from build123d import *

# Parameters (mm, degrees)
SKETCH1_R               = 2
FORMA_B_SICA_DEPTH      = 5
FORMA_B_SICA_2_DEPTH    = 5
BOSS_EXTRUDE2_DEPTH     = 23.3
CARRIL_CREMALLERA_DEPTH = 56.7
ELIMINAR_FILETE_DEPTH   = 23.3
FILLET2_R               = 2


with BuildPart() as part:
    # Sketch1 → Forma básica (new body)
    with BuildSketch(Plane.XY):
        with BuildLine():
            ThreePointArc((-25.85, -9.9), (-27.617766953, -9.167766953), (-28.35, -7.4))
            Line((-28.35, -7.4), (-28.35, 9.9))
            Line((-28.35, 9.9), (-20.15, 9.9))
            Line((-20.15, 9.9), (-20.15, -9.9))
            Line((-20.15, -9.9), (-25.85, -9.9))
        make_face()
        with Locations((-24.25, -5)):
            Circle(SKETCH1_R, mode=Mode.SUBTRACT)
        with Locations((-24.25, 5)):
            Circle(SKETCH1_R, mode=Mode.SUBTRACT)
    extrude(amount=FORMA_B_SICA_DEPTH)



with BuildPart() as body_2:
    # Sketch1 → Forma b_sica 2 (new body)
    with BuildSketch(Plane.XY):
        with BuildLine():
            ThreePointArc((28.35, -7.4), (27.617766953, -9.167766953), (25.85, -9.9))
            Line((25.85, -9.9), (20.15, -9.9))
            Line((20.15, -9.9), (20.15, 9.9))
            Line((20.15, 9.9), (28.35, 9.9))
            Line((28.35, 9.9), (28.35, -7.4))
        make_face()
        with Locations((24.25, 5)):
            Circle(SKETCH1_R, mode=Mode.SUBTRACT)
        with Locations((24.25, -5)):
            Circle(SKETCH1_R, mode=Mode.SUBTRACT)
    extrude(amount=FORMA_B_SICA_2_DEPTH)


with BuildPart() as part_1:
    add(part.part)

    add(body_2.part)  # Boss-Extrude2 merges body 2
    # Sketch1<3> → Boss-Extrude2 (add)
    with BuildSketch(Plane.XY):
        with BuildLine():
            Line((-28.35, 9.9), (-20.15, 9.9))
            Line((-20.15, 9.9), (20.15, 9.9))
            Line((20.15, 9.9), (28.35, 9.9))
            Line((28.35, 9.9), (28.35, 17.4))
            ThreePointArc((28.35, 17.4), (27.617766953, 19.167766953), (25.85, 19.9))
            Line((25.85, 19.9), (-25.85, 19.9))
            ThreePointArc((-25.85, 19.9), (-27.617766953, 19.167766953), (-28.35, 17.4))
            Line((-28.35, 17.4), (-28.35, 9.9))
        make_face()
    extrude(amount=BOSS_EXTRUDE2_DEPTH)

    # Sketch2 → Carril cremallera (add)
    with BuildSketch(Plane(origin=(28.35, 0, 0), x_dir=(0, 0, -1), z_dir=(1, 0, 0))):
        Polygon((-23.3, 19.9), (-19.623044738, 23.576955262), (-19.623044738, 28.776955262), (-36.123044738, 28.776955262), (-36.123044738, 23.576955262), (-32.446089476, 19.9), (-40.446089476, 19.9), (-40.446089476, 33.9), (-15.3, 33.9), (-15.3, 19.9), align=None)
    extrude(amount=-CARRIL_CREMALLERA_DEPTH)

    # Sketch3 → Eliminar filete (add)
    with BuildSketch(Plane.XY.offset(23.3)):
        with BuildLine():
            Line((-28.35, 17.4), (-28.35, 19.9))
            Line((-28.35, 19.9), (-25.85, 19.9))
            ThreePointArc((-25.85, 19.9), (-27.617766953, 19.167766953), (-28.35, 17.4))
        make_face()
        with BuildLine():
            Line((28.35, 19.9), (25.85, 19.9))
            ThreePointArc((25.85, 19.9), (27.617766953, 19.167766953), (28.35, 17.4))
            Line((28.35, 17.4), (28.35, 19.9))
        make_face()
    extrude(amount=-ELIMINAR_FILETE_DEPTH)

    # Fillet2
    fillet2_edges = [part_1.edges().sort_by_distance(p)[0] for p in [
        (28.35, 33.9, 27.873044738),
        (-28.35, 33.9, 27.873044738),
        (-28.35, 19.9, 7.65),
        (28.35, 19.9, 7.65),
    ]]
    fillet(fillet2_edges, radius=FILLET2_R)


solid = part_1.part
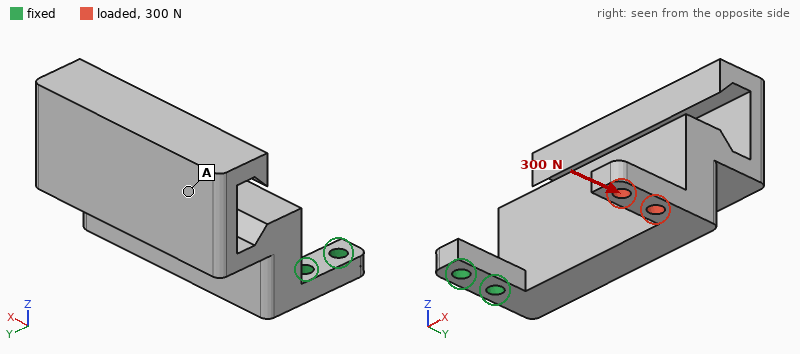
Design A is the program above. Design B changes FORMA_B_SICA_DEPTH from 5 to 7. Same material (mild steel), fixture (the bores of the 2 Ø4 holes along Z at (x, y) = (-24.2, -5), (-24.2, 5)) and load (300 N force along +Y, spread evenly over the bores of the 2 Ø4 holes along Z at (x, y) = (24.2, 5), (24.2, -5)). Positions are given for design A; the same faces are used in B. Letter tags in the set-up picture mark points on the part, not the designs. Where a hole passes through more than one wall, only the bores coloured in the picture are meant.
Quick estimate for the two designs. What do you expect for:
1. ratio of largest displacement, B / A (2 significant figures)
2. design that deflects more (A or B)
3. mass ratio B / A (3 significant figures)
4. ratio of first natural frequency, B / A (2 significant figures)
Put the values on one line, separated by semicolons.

0.75; A; 1.01; 1.4
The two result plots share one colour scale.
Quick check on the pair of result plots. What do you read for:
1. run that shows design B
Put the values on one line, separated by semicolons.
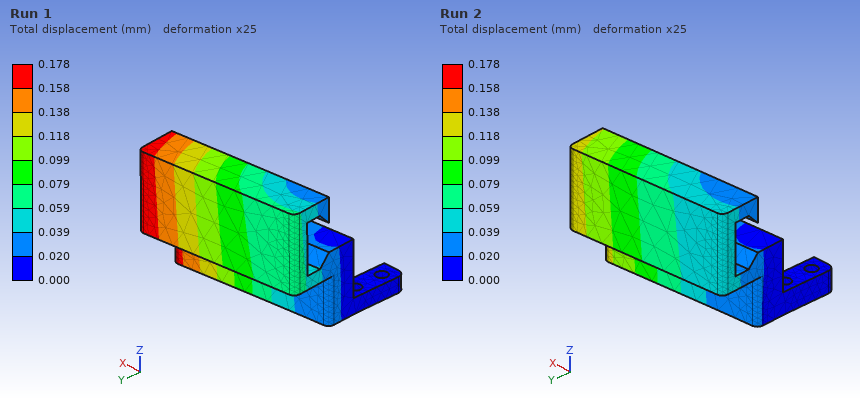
Run 2
